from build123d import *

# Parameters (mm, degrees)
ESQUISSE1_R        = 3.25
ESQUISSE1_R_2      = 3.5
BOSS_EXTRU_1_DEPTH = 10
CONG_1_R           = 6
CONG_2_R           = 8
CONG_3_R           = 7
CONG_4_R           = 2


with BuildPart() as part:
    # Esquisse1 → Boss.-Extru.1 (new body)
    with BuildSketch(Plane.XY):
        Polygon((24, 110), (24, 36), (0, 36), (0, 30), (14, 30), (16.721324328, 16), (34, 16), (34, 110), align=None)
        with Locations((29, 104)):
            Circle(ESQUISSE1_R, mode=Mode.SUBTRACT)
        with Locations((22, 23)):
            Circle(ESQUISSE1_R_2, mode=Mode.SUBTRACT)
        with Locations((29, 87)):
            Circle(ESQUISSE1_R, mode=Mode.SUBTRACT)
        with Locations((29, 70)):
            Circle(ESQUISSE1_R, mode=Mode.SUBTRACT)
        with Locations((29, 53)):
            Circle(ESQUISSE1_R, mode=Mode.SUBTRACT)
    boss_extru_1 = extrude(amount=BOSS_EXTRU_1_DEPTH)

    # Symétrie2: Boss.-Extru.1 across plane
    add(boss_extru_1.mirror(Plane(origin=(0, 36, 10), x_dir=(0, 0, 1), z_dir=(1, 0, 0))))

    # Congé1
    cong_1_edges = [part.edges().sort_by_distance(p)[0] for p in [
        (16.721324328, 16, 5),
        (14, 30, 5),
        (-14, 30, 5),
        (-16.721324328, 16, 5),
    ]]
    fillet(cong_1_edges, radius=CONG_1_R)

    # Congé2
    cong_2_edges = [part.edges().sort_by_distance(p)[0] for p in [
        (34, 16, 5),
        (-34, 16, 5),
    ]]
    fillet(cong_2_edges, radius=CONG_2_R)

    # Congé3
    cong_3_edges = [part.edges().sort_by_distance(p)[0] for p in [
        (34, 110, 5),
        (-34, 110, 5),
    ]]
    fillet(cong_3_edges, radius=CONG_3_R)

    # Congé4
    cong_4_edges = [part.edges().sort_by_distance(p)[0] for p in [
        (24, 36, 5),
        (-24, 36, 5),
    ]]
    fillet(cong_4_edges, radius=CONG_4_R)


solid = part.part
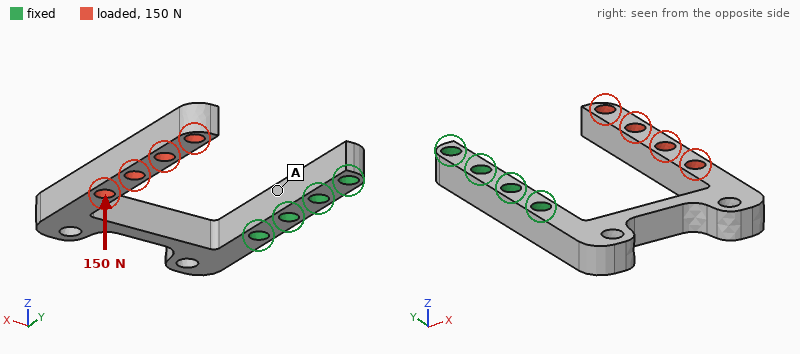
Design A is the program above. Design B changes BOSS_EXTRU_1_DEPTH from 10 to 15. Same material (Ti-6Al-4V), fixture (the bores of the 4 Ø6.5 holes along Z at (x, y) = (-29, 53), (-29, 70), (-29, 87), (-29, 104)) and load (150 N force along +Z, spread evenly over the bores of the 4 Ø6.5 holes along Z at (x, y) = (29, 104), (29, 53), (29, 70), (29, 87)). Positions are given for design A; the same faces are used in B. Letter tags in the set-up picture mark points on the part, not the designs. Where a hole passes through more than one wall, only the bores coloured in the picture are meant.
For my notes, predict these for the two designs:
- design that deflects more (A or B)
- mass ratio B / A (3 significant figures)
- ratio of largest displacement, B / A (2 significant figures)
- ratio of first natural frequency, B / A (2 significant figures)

A
1.50
0.45
1.0
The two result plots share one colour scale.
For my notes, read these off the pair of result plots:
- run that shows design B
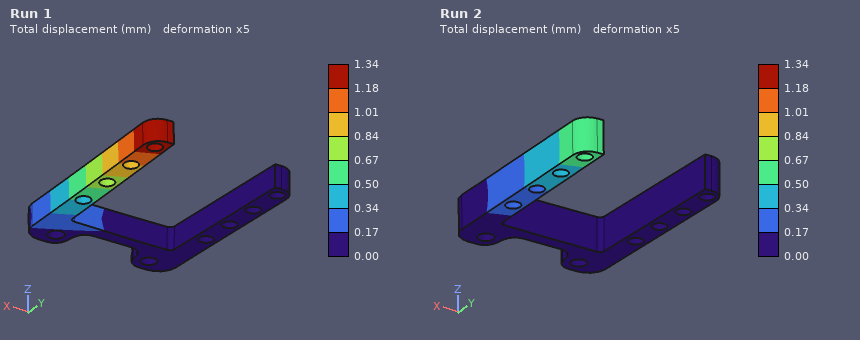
Run 2
